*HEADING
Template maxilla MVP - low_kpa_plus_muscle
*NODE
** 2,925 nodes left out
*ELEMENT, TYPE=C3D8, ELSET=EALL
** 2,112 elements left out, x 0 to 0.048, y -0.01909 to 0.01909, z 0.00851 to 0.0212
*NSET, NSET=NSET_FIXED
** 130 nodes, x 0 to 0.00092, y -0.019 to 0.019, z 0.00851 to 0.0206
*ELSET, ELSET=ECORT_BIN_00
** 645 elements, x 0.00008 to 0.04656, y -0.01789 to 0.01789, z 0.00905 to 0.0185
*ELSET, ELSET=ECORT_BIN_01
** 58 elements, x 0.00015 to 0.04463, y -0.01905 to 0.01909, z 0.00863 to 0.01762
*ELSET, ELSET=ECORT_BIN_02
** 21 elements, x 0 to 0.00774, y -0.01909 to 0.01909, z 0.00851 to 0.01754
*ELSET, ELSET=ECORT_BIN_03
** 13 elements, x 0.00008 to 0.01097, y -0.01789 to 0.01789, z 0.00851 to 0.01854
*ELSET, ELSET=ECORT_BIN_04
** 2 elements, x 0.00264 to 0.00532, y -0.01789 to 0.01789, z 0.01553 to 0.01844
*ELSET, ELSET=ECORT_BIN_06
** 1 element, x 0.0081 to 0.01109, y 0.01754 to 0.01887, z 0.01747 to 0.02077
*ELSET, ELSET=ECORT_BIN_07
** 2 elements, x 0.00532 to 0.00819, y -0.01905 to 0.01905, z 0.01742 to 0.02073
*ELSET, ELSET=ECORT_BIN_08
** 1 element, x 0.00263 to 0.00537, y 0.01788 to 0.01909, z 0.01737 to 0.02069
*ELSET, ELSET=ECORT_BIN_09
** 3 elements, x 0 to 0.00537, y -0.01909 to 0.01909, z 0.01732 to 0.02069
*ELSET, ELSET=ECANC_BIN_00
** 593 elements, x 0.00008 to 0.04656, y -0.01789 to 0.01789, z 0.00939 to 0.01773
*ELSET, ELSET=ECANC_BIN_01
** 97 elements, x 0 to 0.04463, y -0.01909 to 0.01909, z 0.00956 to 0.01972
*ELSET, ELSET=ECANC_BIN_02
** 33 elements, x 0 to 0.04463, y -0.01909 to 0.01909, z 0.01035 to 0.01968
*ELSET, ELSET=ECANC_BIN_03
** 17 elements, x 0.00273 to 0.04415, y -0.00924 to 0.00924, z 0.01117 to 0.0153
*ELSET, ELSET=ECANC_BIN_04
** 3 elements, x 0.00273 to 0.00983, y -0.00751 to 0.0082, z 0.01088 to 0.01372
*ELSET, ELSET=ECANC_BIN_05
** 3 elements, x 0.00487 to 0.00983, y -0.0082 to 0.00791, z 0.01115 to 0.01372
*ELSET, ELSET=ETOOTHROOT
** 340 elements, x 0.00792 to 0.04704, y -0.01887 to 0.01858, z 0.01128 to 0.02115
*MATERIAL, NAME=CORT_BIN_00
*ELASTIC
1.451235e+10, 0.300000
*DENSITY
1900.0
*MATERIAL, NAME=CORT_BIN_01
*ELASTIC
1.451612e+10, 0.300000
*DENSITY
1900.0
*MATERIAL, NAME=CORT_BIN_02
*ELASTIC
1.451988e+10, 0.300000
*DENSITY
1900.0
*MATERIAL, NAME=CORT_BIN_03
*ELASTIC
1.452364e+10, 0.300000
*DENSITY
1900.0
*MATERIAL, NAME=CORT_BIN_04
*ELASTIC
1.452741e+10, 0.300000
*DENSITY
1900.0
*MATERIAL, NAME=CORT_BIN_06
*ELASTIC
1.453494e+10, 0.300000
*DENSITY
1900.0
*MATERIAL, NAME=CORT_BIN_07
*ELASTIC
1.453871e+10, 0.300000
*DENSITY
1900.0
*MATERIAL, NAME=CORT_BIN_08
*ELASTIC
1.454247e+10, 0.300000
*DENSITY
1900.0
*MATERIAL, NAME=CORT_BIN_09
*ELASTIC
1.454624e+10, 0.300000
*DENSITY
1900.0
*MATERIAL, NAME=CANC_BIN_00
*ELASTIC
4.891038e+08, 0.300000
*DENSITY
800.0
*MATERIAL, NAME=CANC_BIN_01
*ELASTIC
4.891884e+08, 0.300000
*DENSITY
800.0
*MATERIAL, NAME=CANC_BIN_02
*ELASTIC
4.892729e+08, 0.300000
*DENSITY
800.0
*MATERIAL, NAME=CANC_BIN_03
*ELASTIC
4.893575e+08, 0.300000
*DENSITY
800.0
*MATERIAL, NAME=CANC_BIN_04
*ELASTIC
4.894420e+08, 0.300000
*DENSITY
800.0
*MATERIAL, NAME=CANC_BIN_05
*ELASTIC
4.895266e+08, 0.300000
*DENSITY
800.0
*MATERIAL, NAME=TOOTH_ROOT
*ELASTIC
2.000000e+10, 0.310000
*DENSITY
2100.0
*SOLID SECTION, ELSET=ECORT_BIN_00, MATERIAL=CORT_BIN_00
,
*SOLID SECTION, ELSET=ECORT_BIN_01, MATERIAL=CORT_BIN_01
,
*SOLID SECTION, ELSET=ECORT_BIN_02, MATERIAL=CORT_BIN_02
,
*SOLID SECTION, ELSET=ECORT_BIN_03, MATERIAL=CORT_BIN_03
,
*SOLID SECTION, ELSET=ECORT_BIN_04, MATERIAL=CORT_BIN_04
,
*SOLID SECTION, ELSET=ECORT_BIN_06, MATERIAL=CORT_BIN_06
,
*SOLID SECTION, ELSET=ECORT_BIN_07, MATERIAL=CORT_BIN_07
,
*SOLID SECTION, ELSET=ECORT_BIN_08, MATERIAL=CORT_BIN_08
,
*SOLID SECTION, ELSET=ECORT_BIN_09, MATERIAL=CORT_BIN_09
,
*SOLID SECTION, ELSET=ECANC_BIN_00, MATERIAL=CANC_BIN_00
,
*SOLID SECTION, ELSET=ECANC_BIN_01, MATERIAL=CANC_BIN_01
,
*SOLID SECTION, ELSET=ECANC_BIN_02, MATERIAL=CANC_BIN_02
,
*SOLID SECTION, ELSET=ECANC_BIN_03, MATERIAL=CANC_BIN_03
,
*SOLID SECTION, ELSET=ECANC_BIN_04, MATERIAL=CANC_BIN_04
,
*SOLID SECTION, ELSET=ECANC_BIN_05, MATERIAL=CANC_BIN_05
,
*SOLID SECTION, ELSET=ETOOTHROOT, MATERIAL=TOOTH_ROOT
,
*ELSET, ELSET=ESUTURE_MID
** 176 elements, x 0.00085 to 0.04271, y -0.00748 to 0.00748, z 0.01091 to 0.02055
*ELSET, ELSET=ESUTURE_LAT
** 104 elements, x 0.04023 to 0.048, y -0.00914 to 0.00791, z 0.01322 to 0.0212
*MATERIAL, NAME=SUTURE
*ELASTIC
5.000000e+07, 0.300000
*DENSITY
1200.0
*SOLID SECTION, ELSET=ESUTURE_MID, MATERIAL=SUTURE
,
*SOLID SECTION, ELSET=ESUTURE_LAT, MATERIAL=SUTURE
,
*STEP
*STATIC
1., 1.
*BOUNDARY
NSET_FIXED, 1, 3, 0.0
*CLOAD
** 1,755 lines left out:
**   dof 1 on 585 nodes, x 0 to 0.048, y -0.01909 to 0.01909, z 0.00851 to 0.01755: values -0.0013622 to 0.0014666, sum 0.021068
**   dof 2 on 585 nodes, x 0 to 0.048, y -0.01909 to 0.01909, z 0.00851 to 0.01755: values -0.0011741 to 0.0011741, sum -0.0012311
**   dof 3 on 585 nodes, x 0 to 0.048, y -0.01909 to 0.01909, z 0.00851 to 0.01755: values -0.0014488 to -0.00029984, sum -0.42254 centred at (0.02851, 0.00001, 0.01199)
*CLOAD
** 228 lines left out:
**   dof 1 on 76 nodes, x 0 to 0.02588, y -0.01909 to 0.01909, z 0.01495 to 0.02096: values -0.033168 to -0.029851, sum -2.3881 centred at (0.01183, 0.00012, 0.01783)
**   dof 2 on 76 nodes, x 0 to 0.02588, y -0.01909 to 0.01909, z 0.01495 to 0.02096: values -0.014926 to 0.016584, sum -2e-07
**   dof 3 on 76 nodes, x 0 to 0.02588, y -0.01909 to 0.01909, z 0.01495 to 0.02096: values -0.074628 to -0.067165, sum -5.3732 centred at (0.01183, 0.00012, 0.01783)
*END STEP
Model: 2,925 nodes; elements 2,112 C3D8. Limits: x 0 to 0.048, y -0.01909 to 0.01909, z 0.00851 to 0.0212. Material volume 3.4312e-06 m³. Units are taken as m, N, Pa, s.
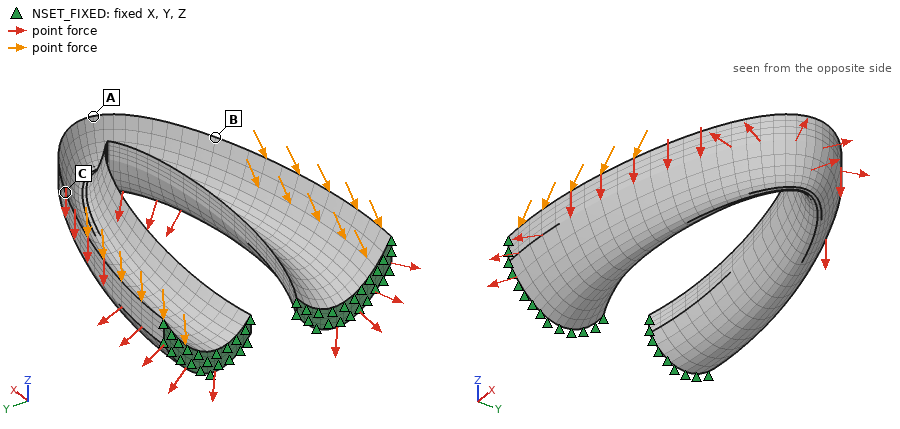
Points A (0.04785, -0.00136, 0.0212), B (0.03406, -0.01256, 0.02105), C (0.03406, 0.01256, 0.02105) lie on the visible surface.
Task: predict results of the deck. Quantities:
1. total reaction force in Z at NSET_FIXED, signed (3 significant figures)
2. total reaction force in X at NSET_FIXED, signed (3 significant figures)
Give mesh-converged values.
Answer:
5.80 N
2.37 N
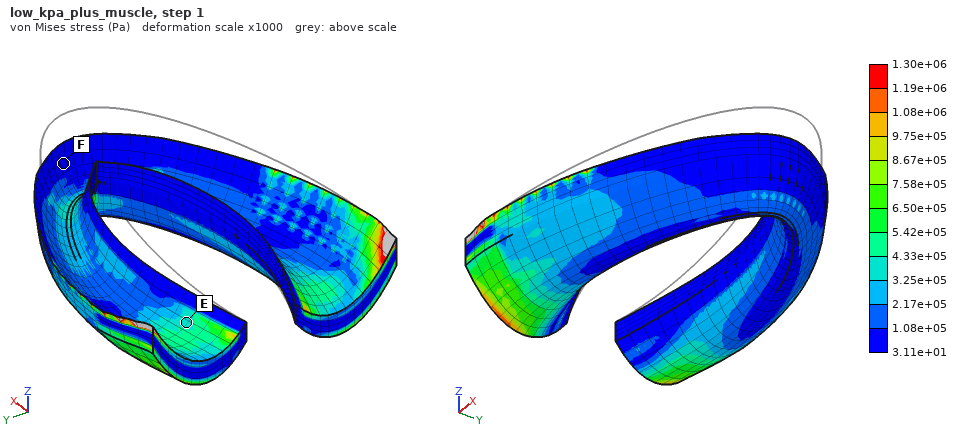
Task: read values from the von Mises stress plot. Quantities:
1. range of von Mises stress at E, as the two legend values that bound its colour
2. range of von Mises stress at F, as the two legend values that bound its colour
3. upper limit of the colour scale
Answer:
3.25e+05 to 4.33e+05 Pa
3.11e+01 to 1.08e+05 Pa
1.30e+06 Pa
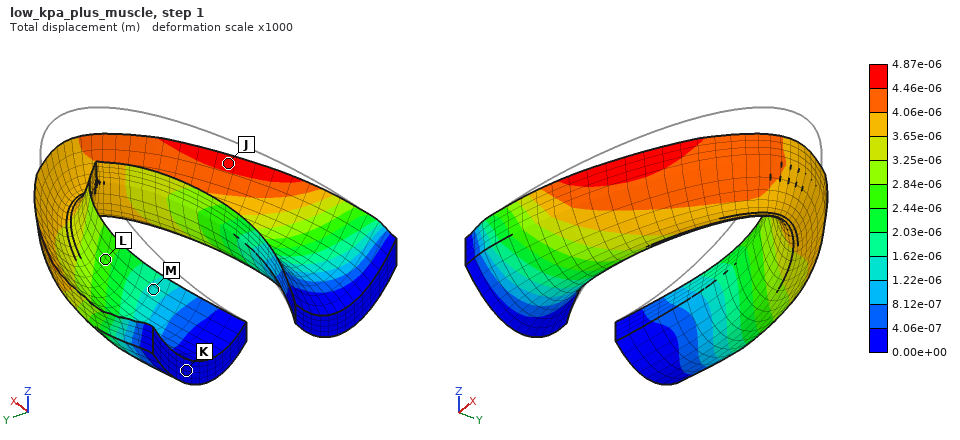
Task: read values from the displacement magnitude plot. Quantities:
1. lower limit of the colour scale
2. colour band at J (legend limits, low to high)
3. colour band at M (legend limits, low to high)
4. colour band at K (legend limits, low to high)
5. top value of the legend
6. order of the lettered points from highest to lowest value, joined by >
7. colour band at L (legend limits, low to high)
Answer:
0.00e+00 m
4.46e-06 to 4.87e-06 m
1.22e-06 to 1.62e-06 m
0.00e+00 to 4.06e-07 m
4.87e-06 m
J > L > M > K
2.44e-06 to 2.84e-06 m
